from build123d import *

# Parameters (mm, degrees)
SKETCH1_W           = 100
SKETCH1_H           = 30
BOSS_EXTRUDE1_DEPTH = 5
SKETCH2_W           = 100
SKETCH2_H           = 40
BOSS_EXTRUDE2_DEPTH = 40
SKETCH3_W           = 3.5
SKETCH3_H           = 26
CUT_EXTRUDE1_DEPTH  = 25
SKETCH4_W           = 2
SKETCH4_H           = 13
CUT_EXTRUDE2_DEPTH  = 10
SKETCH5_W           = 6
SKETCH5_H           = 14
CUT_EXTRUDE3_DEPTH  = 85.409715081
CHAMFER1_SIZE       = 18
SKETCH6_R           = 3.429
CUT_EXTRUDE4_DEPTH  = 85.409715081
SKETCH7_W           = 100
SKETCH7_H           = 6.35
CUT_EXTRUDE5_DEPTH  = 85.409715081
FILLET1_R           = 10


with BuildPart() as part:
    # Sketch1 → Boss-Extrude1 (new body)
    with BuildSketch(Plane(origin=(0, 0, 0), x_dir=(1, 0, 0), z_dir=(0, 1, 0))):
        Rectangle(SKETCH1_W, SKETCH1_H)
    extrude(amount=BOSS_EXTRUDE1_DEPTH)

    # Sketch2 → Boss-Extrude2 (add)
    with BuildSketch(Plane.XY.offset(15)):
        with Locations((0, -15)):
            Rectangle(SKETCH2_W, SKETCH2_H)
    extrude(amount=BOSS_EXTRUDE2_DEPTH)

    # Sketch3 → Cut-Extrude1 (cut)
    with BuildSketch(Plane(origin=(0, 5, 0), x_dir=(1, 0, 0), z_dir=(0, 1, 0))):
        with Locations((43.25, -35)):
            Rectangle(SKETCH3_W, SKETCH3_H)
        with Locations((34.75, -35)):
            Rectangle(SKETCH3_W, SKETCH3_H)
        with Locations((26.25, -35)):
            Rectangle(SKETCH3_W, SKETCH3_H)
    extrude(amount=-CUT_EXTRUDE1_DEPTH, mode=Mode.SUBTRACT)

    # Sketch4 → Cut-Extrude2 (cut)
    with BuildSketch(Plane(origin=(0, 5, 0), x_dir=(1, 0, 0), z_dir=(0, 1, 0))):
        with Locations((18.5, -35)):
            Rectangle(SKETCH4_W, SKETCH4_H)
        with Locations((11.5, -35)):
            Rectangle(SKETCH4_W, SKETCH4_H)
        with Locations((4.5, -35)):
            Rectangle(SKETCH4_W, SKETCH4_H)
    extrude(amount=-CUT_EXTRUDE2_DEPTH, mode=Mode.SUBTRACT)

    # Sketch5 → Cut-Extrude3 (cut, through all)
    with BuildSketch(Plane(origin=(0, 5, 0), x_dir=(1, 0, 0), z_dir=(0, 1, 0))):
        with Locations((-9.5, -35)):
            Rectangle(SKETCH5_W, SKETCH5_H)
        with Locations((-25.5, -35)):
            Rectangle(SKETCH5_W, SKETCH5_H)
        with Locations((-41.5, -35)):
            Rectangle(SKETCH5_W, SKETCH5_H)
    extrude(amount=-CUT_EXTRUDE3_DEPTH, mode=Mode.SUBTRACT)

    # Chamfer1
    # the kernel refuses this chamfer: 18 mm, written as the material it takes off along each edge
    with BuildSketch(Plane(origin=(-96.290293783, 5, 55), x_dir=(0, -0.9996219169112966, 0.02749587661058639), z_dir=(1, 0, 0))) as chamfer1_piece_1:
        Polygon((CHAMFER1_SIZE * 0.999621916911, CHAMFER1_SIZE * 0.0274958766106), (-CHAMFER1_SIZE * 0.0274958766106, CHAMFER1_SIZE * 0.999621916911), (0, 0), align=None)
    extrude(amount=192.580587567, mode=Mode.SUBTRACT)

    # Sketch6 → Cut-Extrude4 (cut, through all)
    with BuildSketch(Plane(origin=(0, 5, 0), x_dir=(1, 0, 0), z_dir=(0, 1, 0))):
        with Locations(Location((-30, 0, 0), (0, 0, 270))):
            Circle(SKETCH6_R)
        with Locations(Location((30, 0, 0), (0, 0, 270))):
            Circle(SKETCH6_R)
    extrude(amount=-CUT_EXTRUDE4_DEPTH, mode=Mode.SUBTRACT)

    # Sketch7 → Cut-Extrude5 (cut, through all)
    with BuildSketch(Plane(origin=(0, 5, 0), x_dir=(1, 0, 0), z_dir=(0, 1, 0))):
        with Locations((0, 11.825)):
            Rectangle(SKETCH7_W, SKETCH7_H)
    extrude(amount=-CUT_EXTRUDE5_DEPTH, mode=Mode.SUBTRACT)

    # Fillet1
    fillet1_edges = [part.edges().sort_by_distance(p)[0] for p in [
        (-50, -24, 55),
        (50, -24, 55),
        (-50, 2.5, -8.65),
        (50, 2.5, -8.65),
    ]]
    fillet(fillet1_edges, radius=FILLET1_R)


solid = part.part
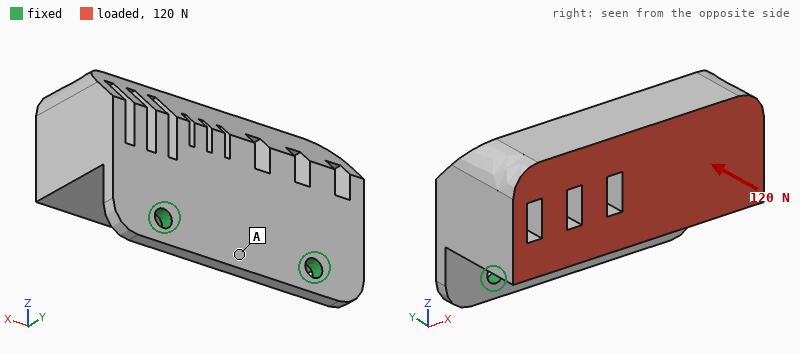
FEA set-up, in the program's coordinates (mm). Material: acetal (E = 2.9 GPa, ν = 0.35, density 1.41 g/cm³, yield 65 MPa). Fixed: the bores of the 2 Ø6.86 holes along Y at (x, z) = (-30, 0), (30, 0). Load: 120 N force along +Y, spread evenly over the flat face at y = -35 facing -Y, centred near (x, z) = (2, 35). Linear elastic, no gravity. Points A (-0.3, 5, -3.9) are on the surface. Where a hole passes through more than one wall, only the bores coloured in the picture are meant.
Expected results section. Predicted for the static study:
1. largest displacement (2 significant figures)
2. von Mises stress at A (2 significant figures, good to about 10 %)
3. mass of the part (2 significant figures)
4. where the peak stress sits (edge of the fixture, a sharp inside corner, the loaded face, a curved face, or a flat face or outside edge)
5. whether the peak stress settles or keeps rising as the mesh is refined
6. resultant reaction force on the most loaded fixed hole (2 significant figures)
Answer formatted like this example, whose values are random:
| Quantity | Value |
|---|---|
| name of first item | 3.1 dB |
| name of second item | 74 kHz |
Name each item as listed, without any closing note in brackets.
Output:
| Quantity | Value |
|---|---|
| largest displacement | 1.2 mm |
| von Mises stress at A | 2.0 MPa |
| mass of the part | 190 g |
| where the peak stress sits | edge of the fixture |
| whether the peak stress settles or keeps rising as the mesh is refined | keeps rising |
| resultant reaction force on the most loaded fixed hole | 63 N |
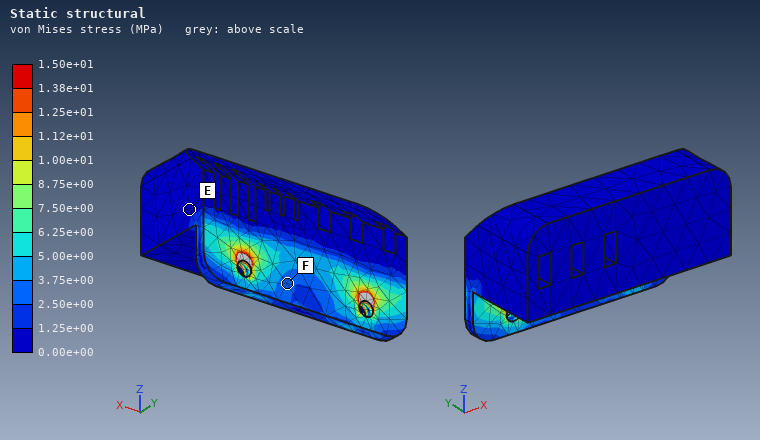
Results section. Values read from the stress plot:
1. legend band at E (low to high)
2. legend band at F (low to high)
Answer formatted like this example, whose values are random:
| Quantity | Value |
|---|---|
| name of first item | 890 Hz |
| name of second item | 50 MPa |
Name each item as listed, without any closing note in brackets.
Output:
| Quantity | Value |
|---|---|
| legend band at E | 0.00e+00 to 1.25e+00 MPa |
| legend band at F | 2.50e+00 to 3.75e+00 MPa |
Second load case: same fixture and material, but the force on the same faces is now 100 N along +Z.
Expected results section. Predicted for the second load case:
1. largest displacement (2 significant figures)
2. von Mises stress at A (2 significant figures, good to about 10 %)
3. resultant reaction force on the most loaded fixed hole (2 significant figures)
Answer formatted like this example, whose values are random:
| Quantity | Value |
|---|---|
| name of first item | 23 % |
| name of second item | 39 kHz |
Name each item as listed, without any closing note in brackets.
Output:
| Quantity | Value |
|---|---|
| largest displacement | 1.4 mm |
| von Mises stress at A | 2.8 MPa |
| resultant reaction force on the most loaded fixed hole | 53 N |
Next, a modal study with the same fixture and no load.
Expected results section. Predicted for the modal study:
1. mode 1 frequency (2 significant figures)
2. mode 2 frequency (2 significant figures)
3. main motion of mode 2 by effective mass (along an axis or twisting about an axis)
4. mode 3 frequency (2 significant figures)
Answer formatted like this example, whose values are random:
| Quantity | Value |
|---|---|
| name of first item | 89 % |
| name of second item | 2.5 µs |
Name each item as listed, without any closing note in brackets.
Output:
| Quantity | Value |
|---|---|
| mode 1 frequency | 130 Hz |
| mode 2 frequency | 590 Hz |
| main motion of mode 2 by effective mass | along X |
| mode 3 frequency | 1000 Hz |
